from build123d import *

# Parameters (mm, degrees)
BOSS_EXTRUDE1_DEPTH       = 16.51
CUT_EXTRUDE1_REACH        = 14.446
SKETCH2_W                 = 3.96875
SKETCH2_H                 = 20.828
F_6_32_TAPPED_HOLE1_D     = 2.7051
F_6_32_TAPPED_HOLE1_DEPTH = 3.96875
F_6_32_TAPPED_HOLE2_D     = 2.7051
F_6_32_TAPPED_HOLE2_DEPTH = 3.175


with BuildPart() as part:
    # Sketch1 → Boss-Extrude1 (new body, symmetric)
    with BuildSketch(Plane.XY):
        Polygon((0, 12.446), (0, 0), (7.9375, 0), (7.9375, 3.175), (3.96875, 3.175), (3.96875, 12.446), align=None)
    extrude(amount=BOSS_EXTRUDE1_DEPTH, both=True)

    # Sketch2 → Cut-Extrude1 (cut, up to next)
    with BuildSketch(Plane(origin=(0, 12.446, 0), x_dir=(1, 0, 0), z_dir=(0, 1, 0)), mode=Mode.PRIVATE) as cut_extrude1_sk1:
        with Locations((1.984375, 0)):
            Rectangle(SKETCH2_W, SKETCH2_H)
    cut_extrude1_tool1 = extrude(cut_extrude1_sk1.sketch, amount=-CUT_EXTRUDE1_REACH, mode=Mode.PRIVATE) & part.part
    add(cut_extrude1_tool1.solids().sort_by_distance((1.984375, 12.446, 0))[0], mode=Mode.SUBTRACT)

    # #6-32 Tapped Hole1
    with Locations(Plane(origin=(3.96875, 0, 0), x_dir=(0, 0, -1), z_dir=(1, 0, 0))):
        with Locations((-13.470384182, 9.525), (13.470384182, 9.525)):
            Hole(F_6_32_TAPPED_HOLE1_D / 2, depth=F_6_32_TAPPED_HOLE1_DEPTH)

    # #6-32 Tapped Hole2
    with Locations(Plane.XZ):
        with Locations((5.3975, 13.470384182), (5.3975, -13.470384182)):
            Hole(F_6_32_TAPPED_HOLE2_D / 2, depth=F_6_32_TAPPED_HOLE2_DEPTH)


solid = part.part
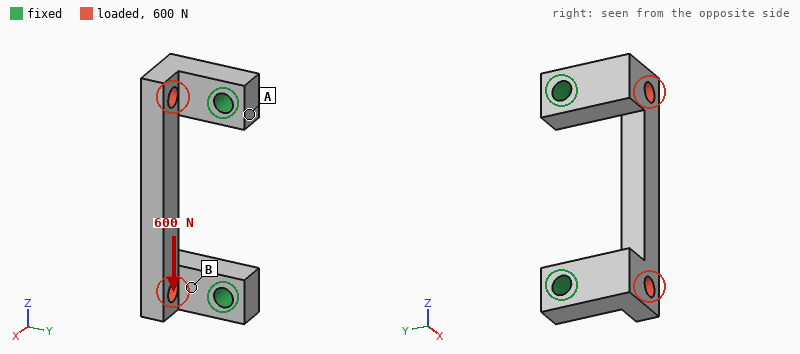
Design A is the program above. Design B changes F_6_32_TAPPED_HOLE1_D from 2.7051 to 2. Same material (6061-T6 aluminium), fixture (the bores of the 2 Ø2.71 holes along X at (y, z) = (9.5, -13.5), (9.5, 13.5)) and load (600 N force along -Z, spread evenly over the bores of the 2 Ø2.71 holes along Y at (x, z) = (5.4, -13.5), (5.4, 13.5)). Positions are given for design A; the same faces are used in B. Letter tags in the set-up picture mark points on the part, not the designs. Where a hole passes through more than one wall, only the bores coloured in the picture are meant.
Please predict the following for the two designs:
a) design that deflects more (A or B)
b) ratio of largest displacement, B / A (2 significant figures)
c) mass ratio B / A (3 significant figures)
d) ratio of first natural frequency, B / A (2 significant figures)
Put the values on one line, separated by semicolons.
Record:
B; 1.2; 1.02; 0.95
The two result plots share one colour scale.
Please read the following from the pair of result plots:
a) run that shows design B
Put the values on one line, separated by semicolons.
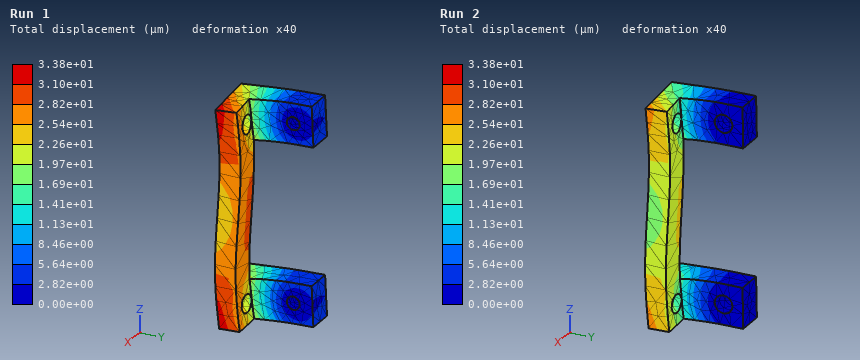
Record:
Run 1
